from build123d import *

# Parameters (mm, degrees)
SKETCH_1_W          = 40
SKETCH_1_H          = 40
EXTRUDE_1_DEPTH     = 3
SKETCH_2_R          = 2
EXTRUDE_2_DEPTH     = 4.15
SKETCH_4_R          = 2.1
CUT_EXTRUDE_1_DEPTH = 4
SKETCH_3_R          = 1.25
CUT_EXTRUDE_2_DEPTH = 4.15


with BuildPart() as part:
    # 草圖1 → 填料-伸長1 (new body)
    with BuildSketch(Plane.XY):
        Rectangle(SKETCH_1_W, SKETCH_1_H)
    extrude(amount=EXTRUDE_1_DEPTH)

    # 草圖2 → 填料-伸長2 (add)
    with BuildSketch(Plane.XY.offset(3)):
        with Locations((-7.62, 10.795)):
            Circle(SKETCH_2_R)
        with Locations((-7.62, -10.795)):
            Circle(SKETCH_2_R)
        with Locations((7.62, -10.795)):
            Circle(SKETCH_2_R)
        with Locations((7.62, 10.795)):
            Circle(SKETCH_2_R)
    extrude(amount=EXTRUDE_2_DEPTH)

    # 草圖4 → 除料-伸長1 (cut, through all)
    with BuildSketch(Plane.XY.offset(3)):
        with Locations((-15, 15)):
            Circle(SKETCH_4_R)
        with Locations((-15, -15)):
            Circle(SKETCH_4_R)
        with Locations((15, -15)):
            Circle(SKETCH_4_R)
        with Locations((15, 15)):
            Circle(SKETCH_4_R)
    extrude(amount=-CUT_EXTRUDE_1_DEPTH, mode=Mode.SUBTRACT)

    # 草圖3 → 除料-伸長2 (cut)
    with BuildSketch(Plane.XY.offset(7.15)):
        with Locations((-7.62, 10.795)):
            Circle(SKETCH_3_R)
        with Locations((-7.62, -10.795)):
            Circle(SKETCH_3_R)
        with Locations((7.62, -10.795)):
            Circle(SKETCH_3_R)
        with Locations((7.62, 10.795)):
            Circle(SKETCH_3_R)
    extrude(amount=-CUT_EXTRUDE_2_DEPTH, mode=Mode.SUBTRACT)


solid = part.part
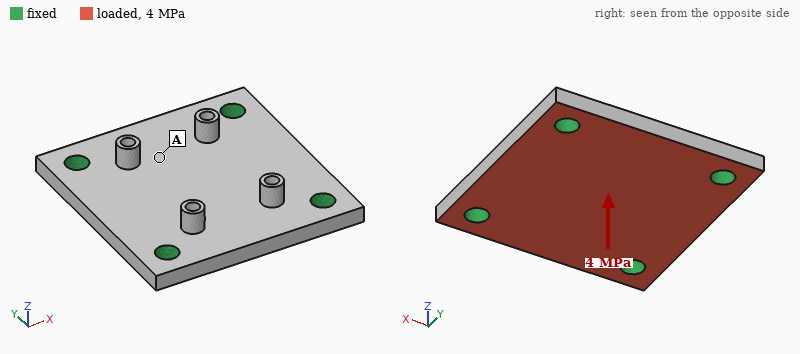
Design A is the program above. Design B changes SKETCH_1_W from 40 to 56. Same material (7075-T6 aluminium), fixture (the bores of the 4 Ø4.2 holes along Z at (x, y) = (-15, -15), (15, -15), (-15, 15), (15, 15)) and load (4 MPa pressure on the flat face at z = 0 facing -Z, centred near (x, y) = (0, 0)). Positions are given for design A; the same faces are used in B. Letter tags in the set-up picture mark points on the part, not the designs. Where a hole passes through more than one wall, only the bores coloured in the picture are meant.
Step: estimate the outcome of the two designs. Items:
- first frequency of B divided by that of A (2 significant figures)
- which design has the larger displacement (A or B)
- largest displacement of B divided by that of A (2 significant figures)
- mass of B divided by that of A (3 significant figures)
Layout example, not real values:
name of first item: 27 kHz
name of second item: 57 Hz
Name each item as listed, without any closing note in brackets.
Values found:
first frequency of B divided by that of A: 0.91
which design has the larger displacement: B
largest displacement of B divided by that of A: 1.3
mass of B divided by that of A: 1.40
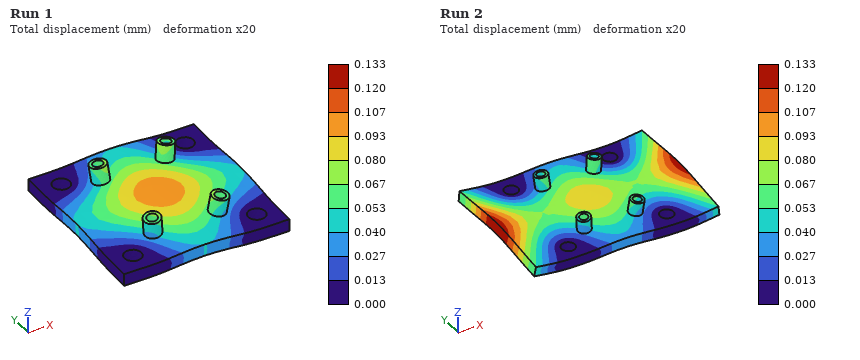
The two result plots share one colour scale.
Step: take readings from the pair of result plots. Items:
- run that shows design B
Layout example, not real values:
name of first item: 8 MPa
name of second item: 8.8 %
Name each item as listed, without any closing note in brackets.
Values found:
run that shows design B: Run 2
